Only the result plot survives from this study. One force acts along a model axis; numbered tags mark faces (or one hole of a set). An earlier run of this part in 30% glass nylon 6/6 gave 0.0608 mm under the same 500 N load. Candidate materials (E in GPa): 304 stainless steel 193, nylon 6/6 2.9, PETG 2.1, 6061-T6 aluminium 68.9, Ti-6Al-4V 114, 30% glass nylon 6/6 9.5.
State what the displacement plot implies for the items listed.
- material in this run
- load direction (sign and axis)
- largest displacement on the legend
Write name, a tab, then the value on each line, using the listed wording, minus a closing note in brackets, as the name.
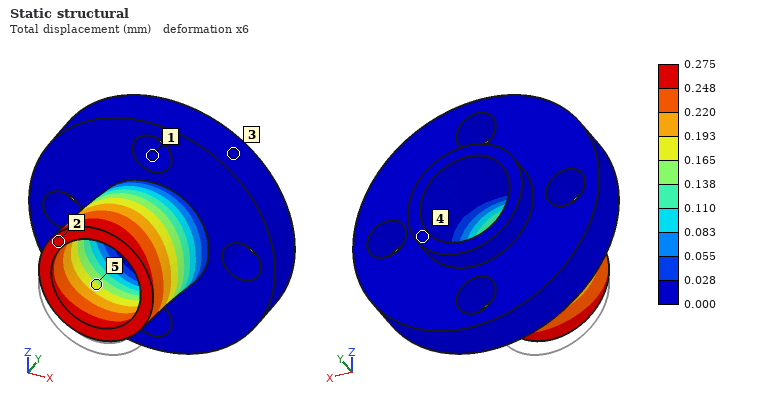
material in this run	PETG
load direction	+Z
largest displacement on the legend	0.275 mm
